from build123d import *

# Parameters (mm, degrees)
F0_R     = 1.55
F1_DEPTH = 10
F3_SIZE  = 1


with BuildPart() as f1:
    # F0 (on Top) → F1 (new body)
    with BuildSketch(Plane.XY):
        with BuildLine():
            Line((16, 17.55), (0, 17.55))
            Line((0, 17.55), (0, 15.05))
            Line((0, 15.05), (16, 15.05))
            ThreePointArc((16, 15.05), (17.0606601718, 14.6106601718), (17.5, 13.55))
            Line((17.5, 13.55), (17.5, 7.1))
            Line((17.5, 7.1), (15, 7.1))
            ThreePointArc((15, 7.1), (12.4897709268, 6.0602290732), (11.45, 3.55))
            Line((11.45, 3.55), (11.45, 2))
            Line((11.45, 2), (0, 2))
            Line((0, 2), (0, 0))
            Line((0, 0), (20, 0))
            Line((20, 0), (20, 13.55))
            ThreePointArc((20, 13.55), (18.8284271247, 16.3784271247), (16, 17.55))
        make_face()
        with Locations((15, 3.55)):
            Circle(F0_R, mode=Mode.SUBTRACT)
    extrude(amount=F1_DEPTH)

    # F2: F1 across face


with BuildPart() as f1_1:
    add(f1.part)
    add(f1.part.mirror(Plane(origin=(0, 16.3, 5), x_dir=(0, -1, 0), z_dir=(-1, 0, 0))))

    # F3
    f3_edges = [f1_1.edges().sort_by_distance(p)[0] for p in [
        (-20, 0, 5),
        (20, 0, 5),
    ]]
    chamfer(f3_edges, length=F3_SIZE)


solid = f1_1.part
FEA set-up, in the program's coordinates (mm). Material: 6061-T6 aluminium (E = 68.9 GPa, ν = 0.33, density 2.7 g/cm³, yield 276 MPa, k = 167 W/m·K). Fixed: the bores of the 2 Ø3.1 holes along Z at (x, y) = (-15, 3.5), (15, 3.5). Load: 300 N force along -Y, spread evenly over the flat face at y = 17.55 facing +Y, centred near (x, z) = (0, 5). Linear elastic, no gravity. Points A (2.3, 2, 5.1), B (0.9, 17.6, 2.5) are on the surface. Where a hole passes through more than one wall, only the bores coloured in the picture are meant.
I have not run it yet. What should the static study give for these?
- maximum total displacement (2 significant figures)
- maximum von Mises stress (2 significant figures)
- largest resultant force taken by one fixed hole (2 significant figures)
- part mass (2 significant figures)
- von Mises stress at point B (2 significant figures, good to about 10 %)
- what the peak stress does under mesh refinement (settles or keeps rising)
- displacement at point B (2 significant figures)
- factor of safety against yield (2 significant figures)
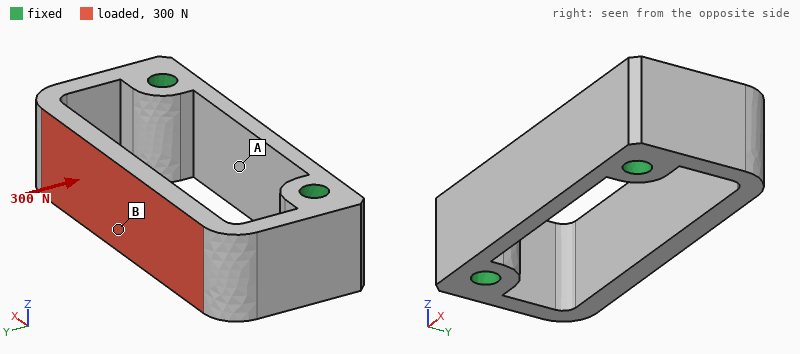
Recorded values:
73 µm
110 MPa
210 N
7.5 g
63 MPa
settles
71 µm
2.5
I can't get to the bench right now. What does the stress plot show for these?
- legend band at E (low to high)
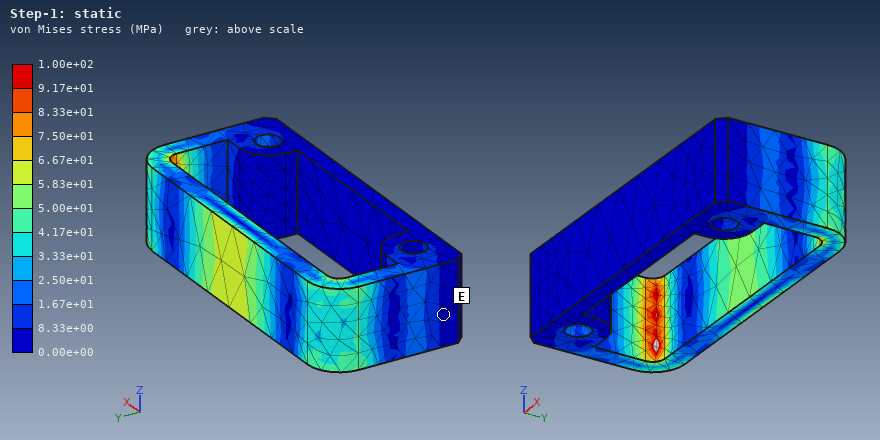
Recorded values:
0.00e+00 to 8.33e+00 MPa
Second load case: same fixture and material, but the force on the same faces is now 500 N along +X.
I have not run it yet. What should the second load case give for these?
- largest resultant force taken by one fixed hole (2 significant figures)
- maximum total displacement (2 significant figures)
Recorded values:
260 N
63 µm
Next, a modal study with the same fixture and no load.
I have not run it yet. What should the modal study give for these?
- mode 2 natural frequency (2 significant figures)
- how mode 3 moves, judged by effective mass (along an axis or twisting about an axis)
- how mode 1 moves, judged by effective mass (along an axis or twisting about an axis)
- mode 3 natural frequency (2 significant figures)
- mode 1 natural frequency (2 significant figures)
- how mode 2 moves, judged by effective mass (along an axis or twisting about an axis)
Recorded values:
8600 Hz
along Z
along Y
11 kHz
7900 Hz
along X
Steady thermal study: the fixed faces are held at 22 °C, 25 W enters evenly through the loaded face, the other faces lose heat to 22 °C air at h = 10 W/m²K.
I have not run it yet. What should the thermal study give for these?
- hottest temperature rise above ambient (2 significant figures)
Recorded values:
62 K
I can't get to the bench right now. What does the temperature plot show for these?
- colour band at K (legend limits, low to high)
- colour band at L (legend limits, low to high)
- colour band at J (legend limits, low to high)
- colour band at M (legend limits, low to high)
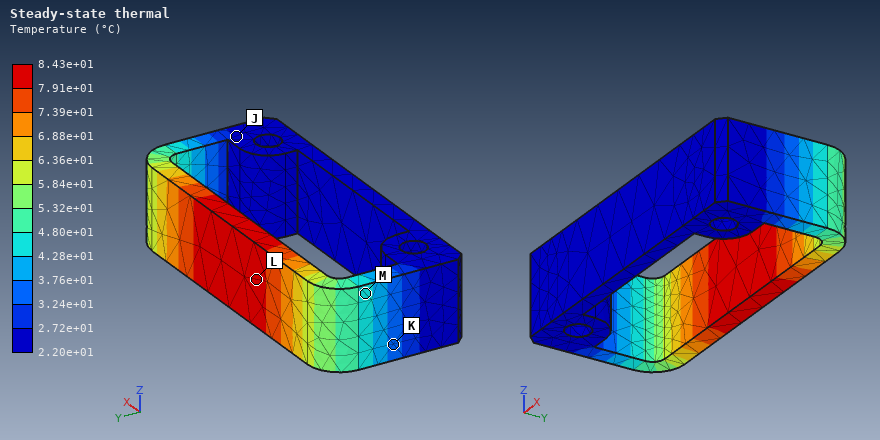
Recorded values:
3.24e+01 to 3.76e+01 °C
7.91e+01 to 8.43e+01 °C
2.20e+01 to 2.72e+01 °C
4.28e+01 to 4.80e+01 °C
